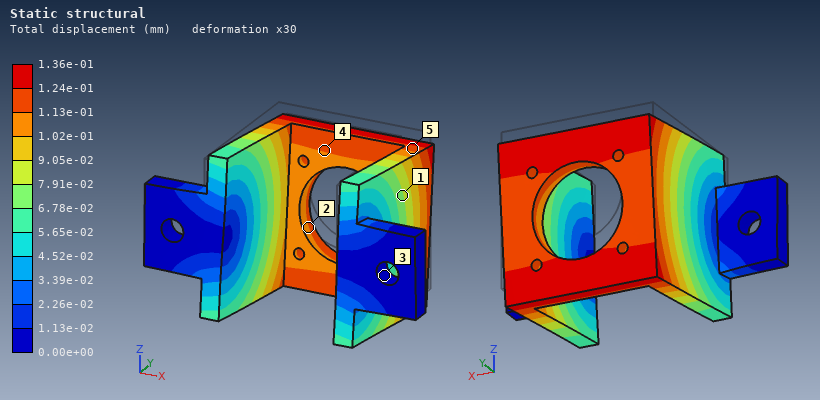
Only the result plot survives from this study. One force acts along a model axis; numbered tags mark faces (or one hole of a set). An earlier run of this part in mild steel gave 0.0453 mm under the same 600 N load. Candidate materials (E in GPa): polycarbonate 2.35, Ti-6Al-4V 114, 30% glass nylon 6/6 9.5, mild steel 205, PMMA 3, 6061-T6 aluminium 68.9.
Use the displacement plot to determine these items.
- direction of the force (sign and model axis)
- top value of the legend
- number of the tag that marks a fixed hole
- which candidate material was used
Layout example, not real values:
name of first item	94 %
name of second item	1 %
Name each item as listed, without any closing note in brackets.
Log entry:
direction of the force	-Z
top value of the legend	1.36e-01 mm
number of the tag that marks a fixed hole	3
which candidate material was used	6061-T6 aluminium
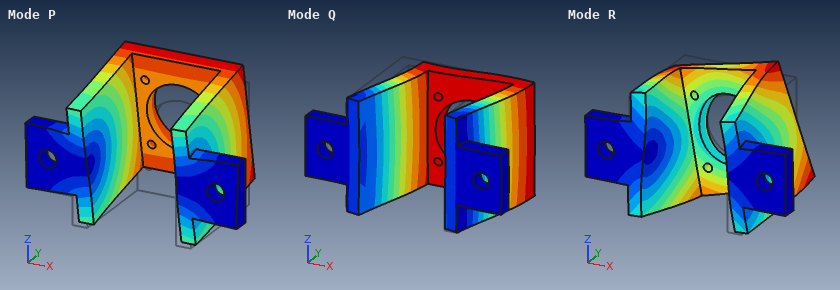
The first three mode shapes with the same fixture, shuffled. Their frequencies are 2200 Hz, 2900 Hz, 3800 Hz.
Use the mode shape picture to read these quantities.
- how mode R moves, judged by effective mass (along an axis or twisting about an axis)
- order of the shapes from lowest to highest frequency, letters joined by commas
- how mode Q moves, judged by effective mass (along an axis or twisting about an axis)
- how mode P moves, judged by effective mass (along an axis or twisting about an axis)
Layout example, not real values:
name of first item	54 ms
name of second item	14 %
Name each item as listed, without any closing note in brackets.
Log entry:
how mode R moves, judged by effective mass	twisting about Y
order of the shapes from lowest to highest frequency, letters joined by commas	P, Q, R
how mode Q moves, judged by effective mass	along X
how mode P moves, judged by effective mass	along Z
